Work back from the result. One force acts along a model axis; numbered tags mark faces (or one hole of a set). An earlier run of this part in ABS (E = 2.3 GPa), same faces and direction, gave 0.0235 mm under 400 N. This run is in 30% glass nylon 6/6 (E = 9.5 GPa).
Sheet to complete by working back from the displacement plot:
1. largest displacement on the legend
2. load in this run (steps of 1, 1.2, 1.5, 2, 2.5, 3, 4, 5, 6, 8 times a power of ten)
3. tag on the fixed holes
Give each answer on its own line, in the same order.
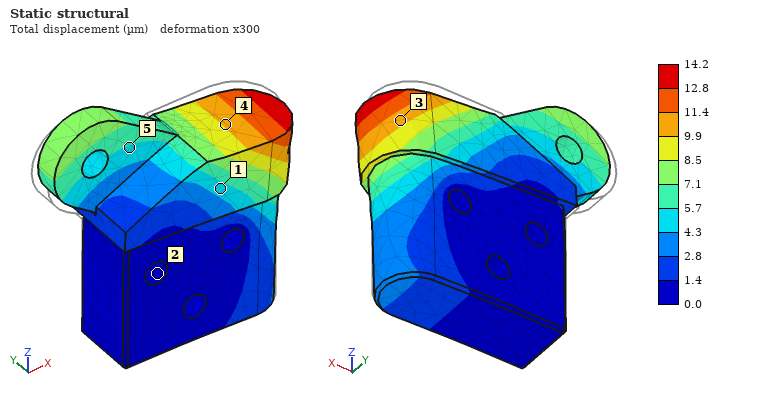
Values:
14.2 µm
1 kN
2
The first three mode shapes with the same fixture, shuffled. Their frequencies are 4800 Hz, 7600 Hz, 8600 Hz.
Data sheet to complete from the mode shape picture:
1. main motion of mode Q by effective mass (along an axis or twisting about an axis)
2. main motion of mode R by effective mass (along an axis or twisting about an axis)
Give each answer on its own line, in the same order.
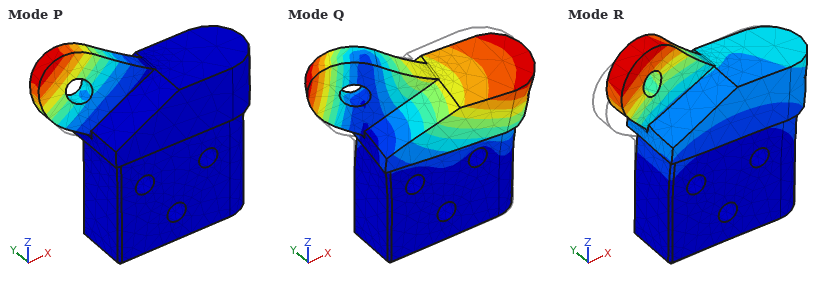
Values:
along Y
along X
